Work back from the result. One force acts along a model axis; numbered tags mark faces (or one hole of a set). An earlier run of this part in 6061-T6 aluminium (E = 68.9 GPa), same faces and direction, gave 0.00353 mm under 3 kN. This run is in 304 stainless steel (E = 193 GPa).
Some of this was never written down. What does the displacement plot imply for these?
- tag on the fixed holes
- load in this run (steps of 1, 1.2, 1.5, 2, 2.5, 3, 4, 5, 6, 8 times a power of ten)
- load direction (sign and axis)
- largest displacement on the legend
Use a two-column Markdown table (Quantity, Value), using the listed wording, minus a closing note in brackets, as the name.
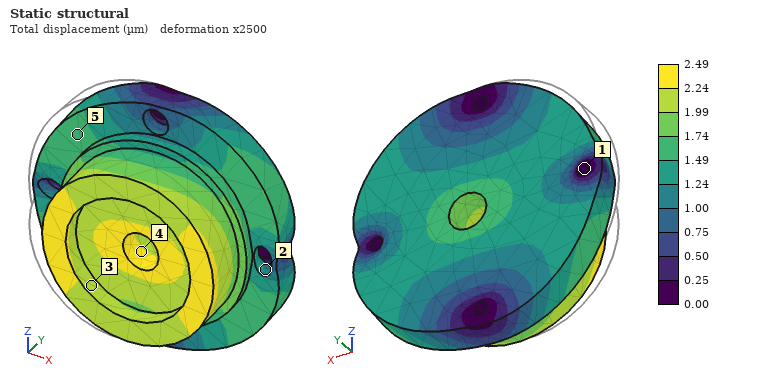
| Quantity | Value |
|---|---|
| tag on the fixed holes | 1 |
| load in this run | 6 kN |
| load direction | +X |
| largest displacement on the legend | 2.49 µm |
